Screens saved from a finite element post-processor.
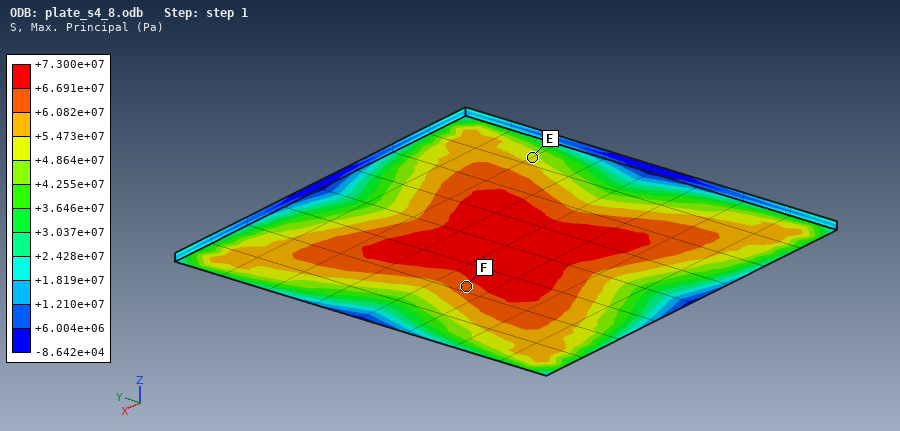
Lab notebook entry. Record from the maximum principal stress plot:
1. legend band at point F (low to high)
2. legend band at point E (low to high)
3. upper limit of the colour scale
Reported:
+6.082e+07 to +6.691e+07 Pa
+4.864e+07 to +5.473e+07 Pa
+7.300e+07 Pa
